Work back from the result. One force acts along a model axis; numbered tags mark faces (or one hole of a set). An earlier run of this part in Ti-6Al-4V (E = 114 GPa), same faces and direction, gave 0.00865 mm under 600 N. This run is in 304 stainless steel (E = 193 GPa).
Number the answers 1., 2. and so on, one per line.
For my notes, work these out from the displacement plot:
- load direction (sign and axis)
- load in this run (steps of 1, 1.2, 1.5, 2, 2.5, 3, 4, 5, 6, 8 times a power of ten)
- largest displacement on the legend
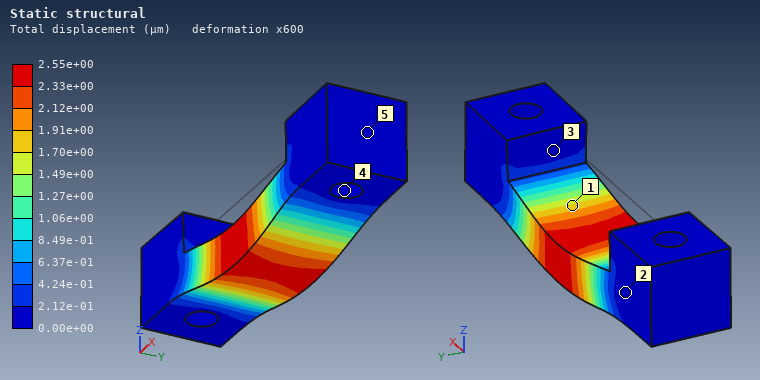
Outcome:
1. -Z
2. 300 N
3. 2.55e+00 µm
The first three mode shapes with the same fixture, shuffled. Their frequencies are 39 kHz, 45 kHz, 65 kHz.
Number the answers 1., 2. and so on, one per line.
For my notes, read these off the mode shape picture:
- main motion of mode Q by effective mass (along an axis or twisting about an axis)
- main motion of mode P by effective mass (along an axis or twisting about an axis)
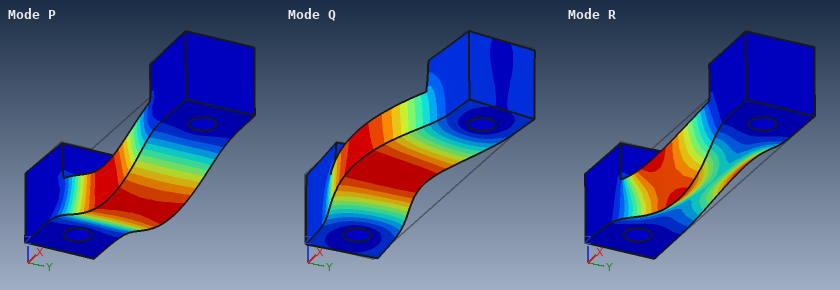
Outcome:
1. along Y
2. along Z
